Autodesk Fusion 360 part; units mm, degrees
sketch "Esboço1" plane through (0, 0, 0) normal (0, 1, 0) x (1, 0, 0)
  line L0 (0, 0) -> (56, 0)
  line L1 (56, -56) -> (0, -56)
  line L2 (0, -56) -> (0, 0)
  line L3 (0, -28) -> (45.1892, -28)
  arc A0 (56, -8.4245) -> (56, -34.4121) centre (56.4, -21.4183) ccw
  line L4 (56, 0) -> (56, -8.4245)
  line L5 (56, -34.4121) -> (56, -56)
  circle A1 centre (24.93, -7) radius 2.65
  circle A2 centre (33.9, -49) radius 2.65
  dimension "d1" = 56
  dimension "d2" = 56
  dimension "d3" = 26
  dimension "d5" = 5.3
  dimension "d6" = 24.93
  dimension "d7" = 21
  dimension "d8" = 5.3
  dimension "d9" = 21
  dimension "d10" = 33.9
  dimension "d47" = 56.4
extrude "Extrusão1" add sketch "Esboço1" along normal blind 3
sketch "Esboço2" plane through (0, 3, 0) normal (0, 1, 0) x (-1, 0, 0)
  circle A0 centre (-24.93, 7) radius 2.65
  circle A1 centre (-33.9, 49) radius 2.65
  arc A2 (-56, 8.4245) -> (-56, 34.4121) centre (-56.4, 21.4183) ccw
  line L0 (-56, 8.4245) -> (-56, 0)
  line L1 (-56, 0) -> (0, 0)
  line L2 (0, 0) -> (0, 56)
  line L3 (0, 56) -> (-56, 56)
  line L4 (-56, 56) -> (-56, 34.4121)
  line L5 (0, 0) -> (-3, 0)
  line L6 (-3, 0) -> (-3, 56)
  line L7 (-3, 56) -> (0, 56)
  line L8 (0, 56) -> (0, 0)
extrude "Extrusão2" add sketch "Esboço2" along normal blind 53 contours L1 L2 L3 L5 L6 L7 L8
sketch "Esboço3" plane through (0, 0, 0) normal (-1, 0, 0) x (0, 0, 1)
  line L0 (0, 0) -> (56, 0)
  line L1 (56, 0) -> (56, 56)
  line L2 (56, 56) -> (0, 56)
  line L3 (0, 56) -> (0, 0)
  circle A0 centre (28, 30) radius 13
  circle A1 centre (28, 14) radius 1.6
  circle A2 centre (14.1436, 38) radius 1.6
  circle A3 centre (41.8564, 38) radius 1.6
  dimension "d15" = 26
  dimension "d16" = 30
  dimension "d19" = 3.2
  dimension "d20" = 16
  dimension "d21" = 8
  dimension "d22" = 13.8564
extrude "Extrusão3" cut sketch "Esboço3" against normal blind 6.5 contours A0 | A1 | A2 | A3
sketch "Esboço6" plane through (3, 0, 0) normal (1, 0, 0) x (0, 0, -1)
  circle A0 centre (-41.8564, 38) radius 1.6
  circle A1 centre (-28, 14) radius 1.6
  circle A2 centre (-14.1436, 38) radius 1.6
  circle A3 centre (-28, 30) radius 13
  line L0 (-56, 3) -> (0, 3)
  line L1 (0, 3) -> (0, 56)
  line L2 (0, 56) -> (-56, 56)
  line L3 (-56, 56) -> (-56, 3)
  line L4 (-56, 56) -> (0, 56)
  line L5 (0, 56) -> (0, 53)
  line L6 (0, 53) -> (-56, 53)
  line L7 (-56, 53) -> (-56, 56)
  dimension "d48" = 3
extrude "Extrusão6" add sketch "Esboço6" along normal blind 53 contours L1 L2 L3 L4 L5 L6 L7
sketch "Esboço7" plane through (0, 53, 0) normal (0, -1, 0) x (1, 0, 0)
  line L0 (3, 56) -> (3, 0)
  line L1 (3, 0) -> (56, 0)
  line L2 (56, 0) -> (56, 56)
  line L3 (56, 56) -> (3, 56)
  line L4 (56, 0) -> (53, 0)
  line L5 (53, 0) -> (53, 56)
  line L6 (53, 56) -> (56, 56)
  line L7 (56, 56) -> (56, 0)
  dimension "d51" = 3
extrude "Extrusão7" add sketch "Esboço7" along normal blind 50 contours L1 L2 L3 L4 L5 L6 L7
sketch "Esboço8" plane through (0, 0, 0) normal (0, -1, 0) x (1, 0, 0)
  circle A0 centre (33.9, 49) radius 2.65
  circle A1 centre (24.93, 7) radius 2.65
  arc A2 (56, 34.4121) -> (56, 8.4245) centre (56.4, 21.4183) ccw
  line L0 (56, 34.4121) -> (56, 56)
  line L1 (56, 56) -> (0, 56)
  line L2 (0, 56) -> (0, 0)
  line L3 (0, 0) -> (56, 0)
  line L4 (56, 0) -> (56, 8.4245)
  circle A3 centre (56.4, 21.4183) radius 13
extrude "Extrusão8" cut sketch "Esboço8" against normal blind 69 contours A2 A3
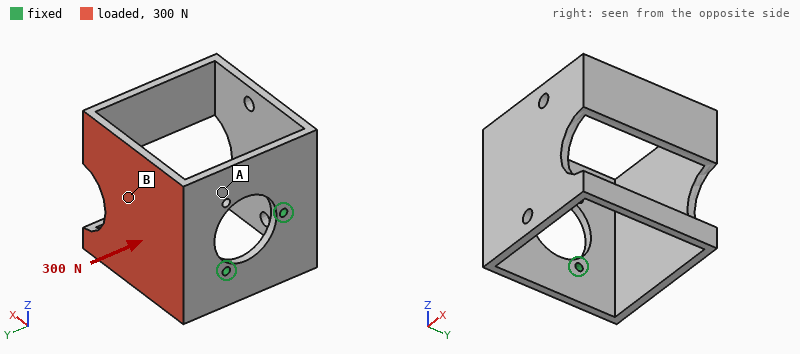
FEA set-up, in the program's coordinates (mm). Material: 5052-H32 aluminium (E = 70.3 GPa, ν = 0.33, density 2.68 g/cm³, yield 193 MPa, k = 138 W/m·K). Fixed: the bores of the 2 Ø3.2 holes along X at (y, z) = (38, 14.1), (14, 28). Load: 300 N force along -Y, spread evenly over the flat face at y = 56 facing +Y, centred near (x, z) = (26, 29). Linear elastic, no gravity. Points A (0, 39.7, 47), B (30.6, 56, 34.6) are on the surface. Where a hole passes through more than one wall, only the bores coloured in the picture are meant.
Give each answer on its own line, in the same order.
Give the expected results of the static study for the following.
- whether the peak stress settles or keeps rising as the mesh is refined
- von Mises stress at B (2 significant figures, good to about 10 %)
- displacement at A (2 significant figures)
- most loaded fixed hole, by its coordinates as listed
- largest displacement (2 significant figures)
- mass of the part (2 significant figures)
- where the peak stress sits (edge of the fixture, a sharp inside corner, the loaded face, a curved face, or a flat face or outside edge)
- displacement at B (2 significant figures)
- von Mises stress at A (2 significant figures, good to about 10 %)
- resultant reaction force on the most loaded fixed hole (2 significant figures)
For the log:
keeps rising
14 MPa
0.090 mm
(14, 28)
0.49 mm
76 g
edge of the fixture
0.33 mm
27 MPa
220 N
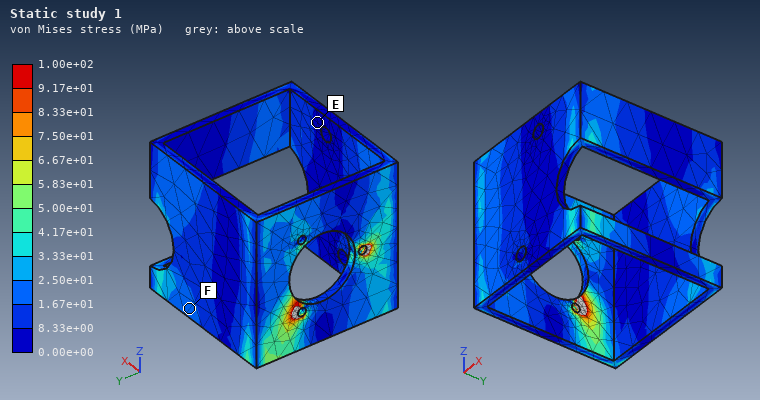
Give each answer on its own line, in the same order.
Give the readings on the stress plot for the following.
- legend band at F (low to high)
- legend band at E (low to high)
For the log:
1.67e+01 to 2.50e+01 MPa
0.00e+00 to 8.33e+00 MPa
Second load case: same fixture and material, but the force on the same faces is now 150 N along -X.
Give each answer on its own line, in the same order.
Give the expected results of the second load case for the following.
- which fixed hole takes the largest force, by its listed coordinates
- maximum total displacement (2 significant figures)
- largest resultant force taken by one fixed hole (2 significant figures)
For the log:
(38, 14.1)
0.27 mm
160 N
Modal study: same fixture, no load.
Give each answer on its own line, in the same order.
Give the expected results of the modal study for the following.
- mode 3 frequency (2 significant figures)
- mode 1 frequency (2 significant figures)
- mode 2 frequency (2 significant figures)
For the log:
1300 Hz
460 Hz
670 Hz
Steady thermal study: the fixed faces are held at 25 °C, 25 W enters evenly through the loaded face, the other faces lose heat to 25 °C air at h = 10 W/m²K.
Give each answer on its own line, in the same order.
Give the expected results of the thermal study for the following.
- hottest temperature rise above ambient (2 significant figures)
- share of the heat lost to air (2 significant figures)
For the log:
44 K
16 %
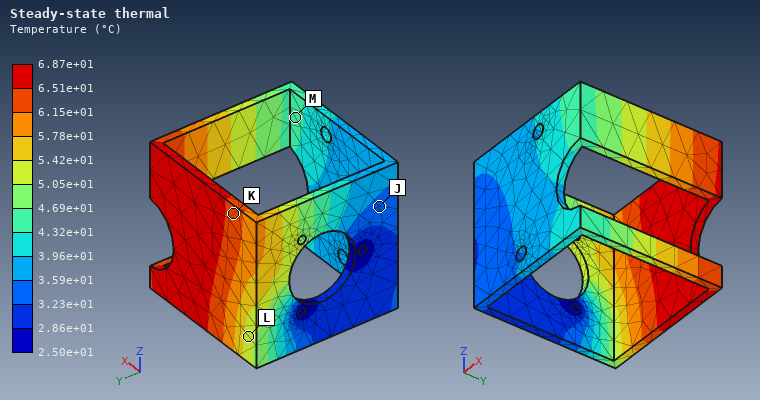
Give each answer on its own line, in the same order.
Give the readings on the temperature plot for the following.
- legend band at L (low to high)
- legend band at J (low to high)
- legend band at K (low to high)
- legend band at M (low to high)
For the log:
5.05e+01 to 5.42e+01 °C
3.23e+01 to 3.59e+01 °C
6.15e+01 to 6.51e+01 °C
4.32e+01 to 4.69e+01 °C
